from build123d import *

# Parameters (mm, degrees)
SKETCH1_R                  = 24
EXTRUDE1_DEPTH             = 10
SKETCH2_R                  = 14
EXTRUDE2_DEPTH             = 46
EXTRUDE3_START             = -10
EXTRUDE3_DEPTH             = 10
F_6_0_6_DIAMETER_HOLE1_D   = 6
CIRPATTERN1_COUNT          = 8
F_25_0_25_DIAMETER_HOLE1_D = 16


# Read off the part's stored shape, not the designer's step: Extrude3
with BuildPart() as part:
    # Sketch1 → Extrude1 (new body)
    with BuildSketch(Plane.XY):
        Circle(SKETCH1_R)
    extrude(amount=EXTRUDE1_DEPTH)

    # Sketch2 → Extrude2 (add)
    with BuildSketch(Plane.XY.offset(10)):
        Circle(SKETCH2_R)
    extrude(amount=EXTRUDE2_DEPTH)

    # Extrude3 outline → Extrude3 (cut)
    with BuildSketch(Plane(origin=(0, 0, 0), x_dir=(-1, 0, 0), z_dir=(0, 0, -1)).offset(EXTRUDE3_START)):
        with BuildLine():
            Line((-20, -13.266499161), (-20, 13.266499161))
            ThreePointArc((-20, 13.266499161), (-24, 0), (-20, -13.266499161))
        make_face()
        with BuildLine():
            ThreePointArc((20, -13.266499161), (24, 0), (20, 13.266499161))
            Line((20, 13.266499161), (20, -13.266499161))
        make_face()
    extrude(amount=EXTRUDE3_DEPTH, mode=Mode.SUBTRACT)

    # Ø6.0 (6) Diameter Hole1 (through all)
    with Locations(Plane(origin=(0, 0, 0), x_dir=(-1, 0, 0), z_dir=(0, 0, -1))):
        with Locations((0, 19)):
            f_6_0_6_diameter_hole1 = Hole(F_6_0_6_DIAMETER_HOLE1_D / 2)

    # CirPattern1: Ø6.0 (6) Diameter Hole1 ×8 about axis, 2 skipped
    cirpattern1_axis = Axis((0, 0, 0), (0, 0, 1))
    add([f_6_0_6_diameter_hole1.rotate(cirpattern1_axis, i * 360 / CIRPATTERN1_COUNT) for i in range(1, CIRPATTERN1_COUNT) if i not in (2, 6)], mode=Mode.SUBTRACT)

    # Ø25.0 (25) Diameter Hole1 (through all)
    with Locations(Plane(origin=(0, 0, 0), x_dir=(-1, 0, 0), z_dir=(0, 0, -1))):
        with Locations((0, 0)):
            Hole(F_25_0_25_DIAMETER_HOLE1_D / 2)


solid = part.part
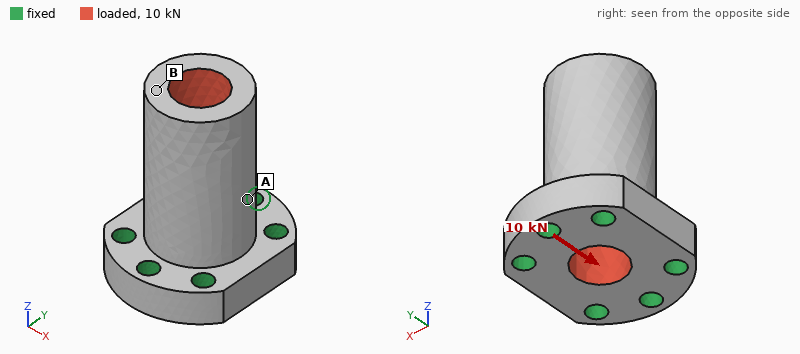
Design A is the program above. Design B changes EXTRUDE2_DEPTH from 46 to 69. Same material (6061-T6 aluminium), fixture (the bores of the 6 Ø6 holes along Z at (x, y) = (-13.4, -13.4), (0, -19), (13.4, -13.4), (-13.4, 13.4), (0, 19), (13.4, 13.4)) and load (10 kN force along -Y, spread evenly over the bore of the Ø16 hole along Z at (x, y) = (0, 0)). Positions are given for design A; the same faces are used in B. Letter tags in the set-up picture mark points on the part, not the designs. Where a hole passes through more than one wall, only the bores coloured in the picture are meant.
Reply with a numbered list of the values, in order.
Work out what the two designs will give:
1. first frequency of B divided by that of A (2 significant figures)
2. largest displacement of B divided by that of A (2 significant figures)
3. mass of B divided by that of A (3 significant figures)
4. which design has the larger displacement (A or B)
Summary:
1. 0.53
2. 2.7
3. 1.30
4. B
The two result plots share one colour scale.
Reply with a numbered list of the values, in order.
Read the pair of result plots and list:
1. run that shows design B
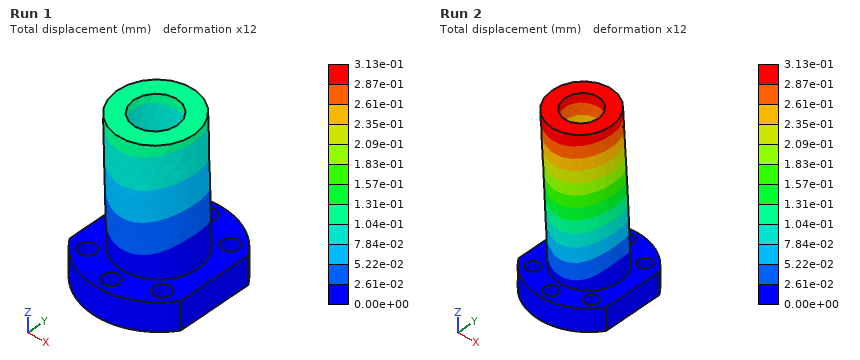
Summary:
1. Run 2
